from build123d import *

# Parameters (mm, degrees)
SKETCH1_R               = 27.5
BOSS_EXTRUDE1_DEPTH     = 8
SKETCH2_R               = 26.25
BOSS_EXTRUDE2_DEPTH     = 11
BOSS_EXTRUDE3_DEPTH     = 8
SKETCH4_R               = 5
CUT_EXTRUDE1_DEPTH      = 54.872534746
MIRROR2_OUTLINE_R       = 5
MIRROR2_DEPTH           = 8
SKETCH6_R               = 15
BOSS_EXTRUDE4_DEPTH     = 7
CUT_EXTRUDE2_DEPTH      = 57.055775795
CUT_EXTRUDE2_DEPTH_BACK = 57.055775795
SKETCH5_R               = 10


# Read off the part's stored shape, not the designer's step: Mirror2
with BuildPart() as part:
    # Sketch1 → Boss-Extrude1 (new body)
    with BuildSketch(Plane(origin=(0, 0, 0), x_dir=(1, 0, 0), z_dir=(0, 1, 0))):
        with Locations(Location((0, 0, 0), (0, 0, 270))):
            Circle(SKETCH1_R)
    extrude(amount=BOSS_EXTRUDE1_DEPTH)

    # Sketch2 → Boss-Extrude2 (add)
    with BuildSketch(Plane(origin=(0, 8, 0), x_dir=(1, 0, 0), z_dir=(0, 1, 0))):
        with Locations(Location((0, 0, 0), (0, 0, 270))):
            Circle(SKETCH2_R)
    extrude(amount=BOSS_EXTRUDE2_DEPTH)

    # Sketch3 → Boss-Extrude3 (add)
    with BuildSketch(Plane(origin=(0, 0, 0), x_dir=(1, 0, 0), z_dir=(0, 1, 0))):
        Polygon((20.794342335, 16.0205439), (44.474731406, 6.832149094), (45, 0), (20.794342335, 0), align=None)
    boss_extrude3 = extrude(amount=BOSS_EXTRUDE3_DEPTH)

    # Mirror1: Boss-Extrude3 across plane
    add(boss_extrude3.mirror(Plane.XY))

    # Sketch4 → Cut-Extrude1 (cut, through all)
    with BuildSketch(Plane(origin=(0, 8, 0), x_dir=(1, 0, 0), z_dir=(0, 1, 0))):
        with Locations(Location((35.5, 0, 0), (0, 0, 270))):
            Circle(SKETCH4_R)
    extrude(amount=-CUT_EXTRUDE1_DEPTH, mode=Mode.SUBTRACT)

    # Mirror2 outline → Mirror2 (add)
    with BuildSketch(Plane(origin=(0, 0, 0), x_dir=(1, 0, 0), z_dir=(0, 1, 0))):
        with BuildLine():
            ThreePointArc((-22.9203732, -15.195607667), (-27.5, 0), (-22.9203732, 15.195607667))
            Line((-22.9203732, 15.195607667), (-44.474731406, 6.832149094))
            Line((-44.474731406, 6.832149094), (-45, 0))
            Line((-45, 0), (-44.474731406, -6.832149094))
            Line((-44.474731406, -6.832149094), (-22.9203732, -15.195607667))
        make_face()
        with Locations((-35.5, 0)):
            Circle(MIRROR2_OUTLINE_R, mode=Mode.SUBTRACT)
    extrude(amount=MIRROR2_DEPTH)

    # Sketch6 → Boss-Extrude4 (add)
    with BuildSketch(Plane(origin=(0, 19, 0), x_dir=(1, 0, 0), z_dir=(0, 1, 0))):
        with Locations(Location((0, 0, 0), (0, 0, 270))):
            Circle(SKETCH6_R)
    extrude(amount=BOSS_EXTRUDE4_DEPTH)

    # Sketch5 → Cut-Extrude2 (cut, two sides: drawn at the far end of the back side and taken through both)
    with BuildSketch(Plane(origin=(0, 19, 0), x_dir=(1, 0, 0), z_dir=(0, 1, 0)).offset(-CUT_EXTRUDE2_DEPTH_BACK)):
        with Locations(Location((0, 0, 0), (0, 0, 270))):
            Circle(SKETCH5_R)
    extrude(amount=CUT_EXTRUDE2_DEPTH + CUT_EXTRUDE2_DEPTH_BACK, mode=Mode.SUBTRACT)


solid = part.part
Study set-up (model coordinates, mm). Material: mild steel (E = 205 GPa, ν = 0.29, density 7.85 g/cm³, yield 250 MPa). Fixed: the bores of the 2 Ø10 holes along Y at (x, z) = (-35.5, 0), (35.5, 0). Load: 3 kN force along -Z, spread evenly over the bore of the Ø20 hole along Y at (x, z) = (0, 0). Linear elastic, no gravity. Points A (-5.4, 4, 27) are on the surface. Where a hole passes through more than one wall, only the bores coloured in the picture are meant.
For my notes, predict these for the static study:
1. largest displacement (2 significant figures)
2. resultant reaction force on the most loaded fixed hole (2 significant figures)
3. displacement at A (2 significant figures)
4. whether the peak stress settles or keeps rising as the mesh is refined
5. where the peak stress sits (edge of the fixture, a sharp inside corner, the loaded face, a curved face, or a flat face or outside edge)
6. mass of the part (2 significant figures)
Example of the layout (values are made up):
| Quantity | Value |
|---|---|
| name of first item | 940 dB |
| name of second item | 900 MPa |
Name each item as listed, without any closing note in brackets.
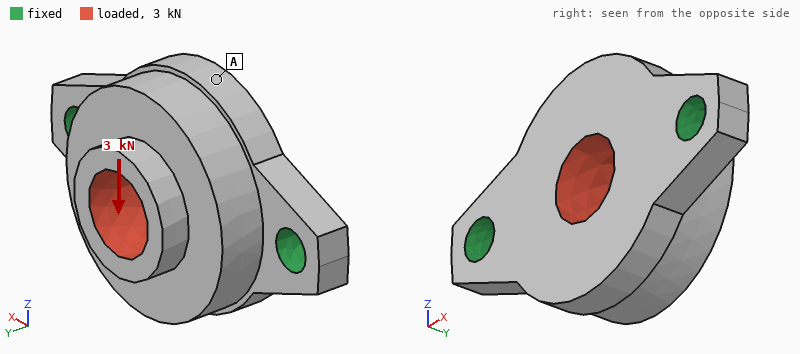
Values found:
| Quantity | Value |
|---|---|
| largest displacement | 12 µm |
| resultant reaction force on the most loaded fixed hole | 1.5 kN |
| displacement at A | 10 µm |
| whether the peak stress settles or keeps rising as the mesh is refined | keeps rising |
| where the peak stress sits | edge of the fixture |
| mass of the part | 350 g |
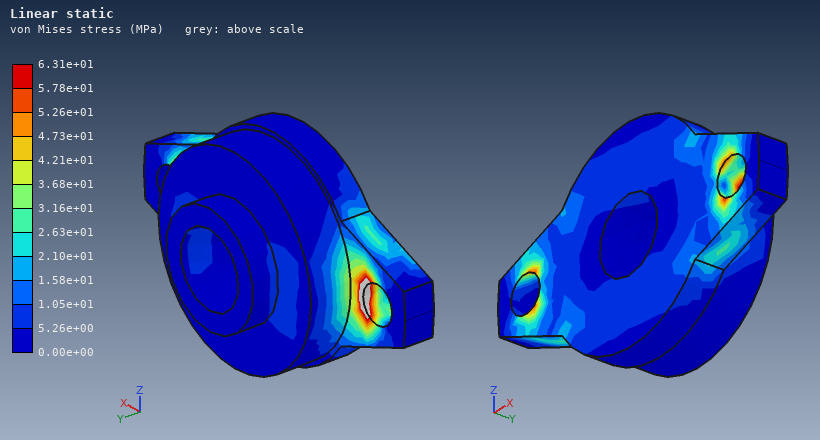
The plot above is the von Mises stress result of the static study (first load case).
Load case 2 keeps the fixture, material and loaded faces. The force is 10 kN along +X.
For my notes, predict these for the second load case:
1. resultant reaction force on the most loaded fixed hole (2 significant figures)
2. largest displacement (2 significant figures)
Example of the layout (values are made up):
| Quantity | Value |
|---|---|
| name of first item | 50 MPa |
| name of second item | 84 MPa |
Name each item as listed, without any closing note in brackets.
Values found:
| Quantity | Value |
|---|---|
| resultant reaction force on the most loaded fixed hole | 5.2 kN |
| largest displacement | 4.9 µm |
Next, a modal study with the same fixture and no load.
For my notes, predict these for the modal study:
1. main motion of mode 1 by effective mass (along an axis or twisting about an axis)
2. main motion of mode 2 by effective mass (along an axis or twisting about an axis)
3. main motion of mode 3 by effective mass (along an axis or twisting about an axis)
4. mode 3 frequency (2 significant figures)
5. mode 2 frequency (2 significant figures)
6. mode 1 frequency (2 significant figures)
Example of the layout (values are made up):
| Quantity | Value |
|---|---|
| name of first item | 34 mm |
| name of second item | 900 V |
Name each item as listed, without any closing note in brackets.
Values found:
| Quantity | Value |
|---|---|
| main motion of mode 1 by effective mass | along Z |
| main motion of mode 2 by effective mass | along Y |
| main motion of mode 3 by effective mass | along Z |
| mode 3 frequency | 14 kHz |
| mode 2 frequency | 8500 Hz |
| mode 1 frequency | 4600 Hz |
